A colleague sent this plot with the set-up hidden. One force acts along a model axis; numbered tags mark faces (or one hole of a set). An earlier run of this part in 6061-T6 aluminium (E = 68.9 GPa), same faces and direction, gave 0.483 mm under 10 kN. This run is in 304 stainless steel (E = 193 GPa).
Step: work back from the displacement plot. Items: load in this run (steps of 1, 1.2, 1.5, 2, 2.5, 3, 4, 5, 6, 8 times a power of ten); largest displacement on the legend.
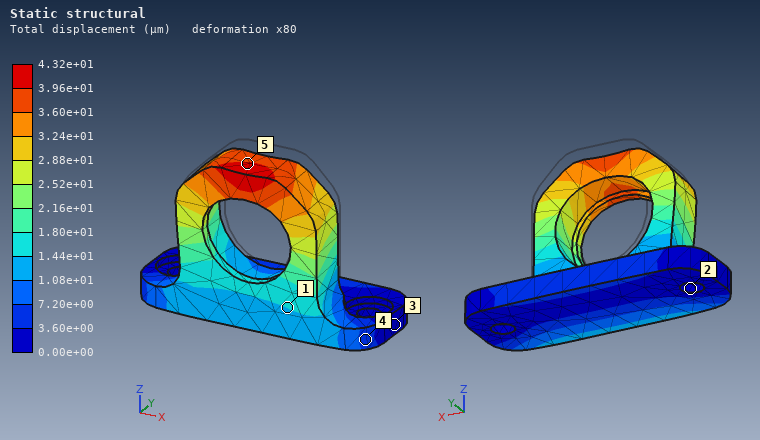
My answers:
2.5 kN
4.32e+01 µm
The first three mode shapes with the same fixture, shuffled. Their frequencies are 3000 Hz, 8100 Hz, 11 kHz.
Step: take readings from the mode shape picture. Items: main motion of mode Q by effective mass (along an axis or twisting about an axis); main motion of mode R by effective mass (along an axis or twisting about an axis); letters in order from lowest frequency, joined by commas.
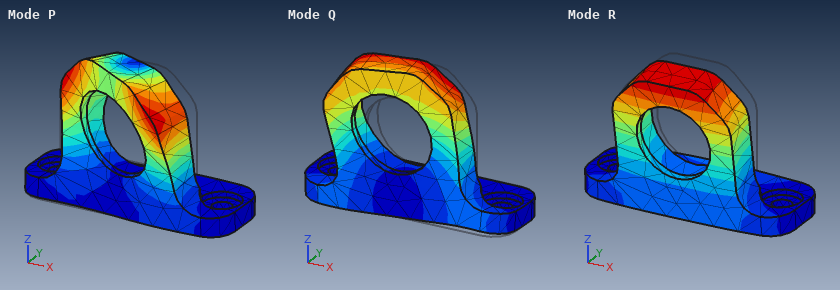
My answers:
along X
along Y
R, Q, P
